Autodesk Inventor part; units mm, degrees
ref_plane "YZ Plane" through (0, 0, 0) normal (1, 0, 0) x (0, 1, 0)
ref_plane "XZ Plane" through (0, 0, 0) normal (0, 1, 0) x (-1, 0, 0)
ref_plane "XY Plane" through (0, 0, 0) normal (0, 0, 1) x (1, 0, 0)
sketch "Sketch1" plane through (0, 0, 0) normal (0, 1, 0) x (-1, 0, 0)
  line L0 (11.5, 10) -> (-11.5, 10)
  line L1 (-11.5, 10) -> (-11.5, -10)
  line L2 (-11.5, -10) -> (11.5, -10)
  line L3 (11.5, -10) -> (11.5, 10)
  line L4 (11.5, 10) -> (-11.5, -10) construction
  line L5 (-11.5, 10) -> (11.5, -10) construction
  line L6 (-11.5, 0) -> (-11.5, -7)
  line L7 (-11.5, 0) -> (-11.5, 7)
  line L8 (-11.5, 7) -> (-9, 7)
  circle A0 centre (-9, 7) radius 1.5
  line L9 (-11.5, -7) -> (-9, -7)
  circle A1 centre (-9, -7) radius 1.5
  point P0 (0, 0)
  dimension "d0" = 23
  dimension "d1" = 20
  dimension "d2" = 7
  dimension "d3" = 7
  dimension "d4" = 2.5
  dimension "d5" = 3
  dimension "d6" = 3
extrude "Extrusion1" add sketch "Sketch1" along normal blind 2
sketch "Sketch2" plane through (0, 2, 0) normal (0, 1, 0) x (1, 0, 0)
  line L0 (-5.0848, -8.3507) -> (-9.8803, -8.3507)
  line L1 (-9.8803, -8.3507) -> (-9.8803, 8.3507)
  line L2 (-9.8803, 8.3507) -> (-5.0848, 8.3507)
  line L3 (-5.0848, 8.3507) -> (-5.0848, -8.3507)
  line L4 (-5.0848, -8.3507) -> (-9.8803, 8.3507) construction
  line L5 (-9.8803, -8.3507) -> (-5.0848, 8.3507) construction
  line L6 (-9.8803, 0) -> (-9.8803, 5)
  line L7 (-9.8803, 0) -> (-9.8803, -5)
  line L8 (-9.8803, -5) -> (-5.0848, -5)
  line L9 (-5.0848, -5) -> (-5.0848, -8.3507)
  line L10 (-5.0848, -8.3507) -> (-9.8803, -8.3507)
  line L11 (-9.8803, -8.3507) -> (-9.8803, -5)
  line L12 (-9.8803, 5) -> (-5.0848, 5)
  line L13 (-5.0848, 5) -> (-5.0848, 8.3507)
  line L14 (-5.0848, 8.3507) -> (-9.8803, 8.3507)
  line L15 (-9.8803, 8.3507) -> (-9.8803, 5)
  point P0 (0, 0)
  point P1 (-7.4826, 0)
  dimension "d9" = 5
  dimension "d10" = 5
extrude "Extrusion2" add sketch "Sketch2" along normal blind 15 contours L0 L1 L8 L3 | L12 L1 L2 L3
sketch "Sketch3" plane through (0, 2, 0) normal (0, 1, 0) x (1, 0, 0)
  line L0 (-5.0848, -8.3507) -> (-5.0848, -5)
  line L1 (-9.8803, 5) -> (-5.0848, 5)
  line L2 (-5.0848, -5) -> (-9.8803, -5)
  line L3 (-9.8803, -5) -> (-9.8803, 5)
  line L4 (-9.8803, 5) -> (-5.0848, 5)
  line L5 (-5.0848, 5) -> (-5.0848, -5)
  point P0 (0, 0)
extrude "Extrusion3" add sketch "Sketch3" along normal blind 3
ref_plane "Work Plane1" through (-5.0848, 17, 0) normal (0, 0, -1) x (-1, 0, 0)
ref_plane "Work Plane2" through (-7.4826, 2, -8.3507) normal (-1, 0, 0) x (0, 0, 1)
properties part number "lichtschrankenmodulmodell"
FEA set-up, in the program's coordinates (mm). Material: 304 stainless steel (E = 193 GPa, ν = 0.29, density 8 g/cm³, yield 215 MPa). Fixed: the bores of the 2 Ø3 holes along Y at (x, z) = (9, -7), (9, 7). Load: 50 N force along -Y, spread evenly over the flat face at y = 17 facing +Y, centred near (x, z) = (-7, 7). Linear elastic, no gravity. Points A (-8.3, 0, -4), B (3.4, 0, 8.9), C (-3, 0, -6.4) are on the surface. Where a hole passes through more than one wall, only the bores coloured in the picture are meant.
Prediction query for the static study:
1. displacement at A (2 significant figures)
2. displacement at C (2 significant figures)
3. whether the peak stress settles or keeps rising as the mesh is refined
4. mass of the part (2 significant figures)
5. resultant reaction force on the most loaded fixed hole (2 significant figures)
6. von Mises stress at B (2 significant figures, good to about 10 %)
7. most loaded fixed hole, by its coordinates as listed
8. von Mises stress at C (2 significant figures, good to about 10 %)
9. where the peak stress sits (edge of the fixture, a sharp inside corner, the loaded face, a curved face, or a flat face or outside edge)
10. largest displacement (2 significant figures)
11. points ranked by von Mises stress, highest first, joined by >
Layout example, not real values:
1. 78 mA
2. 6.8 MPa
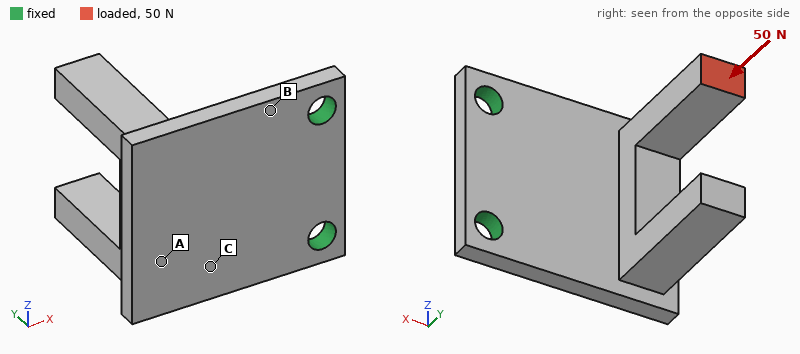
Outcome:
1. 26 µm
2. 13 µm
3. keeps rising
4. 12 g
5. 47 N
6. 53 MPa
7. (9, 7)
8. 23 MPa
9. edge of the fixture
10. 56 µm
11. B > C > A
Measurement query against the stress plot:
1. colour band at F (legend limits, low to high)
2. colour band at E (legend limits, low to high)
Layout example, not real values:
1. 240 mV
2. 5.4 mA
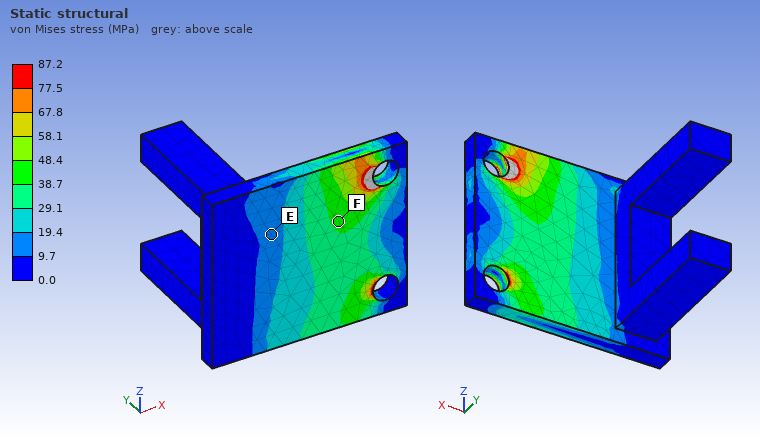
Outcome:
1. 38.7 to 48.4 MPa
2. 9.7 to 19.4 MPa
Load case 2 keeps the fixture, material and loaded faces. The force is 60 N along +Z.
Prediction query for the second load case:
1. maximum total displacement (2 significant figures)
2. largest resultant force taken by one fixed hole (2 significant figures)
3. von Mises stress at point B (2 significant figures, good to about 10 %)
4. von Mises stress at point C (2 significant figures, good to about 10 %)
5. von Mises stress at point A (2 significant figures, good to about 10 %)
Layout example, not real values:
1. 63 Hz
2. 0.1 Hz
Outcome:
1. 52 µm
2. 96 N
3. 40 MPa
4. 31 MPa
5. 16 MPa
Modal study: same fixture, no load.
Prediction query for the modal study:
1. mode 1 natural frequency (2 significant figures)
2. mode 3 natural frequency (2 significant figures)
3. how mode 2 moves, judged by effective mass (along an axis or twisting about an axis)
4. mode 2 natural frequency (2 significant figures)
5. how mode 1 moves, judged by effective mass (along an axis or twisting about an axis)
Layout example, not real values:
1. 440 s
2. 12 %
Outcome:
1. 2000 Hz
2. 8100 Hz
3. along Z
4. 4500 Hz
5. along Y
